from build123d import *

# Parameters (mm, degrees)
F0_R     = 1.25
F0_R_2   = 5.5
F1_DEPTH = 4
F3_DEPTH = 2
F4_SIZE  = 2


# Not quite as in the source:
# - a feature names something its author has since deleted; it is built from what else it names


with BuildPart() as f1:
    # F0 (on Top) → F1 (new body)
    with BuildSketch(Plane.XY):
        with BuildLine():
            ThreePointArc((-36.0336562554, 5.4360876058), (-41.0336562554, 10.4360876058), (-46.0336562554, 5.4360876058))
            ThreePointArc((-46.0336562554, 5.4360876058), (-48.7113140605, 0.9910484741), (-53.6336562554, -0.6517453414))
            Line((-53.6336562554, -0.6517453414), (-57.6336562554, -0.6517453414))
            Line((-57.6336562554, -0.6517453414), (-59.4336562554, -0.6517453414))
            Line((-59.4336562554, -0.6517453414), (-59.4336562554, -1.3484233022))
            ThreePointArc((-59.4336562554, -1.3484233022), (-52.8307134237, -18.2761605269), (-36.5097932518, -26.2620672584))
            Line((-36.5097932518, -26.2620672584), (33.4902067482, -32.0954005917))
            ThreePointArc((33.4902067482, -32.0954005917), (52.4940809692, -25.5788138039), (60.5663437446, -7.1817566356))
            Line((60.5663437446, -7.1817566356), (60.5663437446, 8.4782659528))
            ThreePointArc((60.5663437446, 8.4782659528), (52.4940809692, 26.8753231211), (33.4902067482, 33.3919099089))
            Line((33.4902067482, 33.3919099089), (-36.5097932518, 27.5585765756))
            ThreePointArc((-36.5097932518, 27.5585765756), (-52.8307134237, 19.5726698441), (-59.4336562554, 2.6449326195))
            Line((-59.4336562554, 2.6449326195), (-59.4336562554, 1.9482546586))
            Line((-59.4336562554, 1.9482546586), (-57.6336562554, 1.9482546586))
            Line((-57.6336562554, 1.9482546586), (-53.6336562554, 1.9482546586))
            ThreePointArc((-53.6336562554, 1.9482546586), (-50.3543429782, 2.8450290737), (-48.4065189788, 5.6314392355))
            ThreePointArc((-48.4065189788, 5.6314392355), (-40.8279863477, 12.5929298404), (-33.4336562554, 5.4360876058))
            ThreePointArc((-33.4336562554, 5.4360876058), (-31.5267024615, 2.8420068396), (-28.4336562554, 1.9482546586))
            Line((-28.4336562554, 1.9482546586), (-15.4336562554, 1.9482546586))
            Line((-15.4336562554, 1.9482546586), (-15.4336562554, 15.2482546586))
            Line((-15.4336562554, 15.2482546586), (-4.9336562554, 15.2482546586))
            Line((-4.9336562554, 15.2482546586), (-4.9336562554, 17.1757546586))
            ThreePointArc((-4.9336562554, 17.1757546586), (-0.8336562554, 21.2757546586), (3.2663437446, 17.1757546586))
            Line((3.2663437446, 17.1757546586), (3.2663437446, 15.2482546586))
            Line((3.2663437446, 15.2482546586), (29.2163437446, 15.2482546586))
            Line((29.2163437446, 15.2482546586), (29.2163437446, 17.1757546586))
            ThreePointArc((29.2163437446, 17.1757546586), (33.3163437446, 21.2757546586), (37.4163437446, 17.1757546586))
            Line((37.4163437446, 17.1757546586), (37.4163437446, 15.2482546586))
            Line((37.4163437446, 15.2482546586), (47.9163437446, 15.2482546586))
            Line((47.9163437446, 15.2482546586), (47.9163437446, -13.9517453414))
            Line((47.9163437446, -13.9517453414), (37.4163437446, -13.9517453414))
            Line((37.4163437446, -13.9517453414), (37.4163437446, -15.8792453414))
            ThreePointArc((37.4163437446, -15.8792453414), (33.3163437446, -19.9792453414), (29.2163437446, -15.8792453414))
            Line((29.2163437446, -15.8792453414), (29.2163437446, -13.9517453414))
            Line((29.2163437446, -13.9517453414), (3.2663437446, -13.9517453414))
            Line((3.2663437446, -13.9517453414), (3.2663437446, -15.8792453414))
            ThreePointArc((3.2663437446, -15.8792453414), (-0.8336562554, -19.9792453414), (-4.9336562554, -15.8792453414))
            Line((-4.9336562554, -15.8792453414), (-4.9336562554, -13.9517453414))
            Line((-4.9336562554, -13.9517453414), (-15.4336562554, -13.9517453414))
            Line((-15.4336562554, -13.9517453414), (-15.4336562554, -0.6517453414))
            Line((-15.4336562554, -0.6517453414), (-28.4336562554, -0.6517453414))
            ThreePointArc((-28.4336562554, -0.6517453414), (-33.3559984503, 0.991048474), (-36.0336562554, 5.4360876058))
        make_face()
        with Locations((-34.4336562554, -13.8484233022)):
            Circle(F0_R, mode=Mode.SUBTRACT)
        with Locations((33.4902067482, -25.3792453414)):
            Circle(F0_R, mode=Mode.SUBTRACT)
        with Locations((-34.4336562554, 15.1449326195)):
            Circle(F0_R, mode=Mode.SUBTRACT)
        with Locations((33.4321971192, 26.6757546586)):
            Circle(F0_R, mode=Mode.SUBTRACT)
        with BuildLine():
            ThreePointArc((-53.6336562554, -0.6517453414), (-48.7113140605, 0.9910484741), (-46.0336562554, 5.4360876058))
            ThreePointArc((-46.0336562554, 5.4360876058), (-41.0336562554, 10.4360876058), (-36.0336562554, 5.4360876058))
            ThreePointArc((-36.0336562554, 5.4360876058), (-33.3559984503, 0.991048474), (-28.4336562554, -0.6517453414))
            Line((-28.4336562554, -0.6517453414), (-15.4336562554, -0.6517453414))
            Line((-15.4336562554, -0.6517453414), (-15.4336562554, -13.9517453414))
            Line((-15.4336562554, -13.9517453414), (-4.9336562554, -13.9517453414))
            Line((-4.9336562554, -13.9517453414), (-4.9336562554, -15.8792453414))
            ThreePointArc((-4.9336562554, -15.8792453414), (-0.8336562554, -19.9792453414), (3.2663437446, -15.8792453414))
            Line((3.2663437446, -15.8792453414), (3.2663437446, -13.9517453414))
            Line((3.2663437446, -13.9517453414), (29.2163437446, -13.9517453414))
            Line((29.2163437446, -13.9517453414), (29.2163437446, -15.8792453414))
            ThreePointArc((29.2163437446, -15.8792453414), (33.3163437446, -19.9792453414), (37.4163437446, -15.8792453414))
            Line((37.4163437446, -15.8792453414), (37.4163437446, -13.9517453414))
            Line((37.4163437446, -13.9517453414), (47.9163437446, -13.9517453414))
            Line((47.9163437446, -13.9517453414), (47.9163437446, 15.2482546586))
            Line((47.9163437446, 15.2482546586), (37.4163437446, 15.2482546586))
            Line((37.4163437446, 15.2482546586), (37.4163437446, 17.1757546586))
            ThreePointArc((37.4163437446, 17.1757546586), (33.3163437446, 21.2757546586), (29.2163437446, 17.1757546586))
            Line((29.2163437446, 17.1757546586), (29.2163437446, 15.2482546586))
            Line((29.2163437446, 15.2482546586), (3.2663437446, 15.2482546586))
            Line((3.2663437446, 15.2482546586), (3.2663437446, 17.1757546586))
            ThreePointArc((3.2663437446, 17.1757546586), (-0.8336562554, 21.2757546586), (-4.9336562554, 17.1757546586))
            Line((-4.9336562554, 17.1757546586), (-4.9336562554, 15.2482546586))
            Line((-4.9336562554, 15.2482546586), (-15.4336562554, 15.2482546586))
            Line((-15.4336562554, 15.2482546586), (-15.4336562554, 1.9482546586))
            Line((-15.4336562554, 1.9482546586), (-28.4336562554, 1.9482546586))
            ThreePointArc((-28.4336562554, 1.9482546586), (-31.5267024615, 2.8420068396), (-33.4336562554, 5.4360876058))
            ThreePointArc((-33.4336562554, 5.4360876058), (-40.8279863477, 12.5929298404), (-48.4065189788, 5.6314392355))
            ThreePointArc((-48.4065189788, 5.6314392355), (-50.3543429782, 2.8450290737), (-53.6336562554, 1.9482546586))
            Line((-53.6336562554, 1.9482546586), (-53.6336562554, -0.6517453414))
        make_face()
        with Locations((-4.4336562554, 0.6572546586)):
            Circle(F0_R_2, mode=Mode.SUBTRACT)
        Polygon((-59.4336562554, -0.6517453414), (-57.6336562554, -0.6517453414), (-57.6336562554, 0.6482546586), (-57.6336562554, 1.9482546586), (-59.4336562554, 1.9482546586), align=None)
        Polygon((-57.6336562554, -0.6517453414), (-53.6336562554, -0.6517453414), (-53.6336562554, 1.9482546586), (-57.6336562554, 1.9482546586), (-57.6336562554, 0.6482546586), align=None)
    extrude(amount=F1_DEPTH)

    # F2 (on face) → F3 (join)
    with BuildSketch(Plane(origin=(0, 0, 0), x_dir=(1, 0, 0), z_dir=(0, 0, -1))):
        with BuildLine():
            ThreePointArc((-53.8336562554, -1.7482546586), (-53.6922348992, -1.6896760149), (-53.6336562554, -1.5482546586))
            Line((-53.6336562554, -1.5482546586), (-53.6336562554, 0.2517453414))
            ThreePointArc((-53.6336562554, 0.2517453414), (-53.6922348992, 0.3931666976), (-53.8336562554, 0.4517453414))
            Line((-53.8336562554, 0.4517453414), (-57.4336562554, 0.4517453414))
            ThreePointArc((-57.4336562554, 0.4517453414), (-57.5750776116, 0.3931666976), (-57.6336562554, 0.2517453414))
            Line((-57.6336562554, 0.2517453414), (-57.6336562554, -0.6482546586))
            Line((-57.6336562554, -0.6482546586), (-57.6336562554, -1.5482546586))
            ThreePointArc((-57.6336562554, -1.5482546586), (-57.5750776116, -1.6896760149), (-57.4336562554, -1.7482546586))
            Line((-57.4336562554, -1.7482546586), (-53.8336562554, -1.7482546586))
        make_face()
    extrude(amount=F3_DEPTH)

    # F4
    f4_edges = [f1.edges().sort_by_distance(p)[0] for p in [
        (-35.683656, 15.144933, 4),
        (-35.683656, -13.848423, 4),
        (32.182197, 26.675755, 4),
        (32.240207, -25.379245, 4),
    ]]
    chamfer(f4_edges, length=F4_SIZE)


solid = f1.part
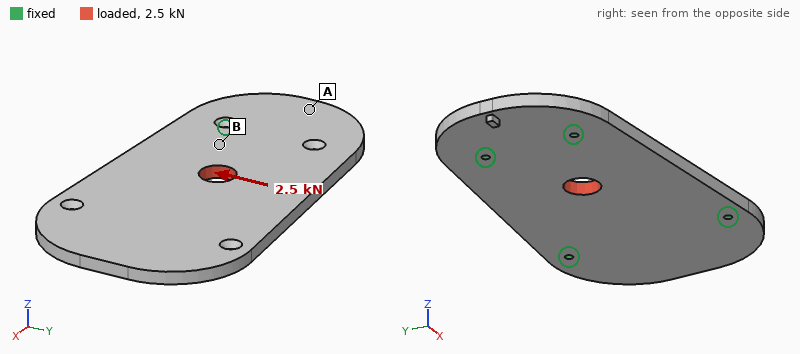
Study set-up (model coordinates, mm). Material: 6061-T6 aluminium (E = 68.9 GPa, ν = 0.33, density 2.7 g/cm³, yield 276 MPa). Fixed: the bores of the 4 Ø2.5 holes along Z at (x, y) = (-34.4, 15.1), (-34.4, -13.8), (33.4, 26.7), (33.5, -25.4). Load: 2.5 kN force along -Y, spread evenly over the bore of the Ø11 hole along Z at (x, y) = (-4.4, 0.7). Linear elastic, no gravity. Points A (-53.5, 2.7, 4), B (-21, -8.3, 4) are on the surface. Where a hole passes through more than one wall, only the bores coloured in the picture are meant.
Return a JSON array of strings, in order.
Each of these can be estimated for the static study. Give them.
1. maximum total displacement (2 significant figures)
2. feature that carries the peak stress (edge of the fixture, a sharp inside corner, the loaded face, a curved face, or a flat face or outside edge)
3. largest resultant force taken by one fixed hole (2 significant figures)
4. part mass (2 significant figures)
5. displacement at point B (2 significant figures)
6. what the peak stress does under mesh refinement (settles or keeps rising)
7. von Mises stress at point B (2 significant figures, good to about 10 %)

["12 µm", "edge of the fixture", "740 N", "70 g", "5.9 µm", "keeps rising", "13 MPa"]
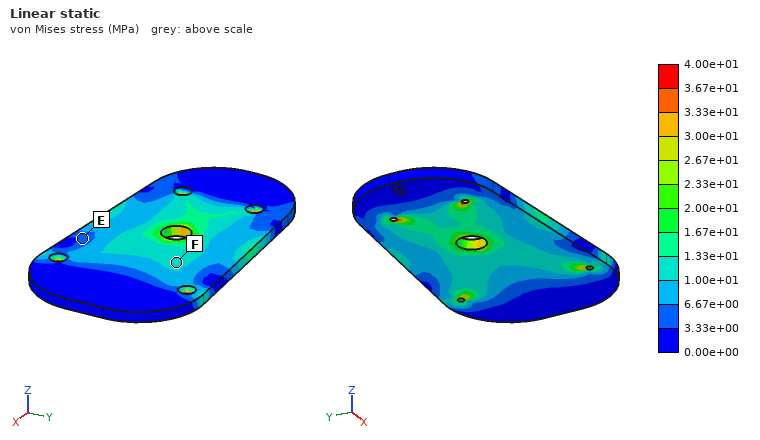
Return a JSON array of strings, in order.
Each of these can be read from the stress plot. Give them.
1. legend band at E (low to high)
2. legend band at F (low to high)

["3.33e+00 to 6.67e+00 MPa", "1.00e+01 to 1.33e+01 MPa"]
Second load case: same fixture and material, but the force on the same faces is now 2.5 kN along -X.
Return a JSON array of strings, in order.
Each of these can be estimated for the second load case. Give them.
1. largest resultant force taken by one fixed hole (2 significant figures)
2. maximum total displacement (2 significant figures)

["700 N", "10 µm"]
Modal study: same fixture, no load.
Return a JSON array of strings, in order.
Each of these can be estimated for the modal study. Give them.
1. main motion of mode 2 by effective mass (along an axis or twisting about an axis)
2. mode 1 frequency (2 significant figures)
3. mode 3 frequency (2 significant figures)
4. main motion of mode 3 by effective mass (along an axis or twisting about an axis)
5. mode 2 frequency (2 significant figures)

["along Z", "2600 Hz", "4400 Hz", "twisting about X", "3200 Hz"]
